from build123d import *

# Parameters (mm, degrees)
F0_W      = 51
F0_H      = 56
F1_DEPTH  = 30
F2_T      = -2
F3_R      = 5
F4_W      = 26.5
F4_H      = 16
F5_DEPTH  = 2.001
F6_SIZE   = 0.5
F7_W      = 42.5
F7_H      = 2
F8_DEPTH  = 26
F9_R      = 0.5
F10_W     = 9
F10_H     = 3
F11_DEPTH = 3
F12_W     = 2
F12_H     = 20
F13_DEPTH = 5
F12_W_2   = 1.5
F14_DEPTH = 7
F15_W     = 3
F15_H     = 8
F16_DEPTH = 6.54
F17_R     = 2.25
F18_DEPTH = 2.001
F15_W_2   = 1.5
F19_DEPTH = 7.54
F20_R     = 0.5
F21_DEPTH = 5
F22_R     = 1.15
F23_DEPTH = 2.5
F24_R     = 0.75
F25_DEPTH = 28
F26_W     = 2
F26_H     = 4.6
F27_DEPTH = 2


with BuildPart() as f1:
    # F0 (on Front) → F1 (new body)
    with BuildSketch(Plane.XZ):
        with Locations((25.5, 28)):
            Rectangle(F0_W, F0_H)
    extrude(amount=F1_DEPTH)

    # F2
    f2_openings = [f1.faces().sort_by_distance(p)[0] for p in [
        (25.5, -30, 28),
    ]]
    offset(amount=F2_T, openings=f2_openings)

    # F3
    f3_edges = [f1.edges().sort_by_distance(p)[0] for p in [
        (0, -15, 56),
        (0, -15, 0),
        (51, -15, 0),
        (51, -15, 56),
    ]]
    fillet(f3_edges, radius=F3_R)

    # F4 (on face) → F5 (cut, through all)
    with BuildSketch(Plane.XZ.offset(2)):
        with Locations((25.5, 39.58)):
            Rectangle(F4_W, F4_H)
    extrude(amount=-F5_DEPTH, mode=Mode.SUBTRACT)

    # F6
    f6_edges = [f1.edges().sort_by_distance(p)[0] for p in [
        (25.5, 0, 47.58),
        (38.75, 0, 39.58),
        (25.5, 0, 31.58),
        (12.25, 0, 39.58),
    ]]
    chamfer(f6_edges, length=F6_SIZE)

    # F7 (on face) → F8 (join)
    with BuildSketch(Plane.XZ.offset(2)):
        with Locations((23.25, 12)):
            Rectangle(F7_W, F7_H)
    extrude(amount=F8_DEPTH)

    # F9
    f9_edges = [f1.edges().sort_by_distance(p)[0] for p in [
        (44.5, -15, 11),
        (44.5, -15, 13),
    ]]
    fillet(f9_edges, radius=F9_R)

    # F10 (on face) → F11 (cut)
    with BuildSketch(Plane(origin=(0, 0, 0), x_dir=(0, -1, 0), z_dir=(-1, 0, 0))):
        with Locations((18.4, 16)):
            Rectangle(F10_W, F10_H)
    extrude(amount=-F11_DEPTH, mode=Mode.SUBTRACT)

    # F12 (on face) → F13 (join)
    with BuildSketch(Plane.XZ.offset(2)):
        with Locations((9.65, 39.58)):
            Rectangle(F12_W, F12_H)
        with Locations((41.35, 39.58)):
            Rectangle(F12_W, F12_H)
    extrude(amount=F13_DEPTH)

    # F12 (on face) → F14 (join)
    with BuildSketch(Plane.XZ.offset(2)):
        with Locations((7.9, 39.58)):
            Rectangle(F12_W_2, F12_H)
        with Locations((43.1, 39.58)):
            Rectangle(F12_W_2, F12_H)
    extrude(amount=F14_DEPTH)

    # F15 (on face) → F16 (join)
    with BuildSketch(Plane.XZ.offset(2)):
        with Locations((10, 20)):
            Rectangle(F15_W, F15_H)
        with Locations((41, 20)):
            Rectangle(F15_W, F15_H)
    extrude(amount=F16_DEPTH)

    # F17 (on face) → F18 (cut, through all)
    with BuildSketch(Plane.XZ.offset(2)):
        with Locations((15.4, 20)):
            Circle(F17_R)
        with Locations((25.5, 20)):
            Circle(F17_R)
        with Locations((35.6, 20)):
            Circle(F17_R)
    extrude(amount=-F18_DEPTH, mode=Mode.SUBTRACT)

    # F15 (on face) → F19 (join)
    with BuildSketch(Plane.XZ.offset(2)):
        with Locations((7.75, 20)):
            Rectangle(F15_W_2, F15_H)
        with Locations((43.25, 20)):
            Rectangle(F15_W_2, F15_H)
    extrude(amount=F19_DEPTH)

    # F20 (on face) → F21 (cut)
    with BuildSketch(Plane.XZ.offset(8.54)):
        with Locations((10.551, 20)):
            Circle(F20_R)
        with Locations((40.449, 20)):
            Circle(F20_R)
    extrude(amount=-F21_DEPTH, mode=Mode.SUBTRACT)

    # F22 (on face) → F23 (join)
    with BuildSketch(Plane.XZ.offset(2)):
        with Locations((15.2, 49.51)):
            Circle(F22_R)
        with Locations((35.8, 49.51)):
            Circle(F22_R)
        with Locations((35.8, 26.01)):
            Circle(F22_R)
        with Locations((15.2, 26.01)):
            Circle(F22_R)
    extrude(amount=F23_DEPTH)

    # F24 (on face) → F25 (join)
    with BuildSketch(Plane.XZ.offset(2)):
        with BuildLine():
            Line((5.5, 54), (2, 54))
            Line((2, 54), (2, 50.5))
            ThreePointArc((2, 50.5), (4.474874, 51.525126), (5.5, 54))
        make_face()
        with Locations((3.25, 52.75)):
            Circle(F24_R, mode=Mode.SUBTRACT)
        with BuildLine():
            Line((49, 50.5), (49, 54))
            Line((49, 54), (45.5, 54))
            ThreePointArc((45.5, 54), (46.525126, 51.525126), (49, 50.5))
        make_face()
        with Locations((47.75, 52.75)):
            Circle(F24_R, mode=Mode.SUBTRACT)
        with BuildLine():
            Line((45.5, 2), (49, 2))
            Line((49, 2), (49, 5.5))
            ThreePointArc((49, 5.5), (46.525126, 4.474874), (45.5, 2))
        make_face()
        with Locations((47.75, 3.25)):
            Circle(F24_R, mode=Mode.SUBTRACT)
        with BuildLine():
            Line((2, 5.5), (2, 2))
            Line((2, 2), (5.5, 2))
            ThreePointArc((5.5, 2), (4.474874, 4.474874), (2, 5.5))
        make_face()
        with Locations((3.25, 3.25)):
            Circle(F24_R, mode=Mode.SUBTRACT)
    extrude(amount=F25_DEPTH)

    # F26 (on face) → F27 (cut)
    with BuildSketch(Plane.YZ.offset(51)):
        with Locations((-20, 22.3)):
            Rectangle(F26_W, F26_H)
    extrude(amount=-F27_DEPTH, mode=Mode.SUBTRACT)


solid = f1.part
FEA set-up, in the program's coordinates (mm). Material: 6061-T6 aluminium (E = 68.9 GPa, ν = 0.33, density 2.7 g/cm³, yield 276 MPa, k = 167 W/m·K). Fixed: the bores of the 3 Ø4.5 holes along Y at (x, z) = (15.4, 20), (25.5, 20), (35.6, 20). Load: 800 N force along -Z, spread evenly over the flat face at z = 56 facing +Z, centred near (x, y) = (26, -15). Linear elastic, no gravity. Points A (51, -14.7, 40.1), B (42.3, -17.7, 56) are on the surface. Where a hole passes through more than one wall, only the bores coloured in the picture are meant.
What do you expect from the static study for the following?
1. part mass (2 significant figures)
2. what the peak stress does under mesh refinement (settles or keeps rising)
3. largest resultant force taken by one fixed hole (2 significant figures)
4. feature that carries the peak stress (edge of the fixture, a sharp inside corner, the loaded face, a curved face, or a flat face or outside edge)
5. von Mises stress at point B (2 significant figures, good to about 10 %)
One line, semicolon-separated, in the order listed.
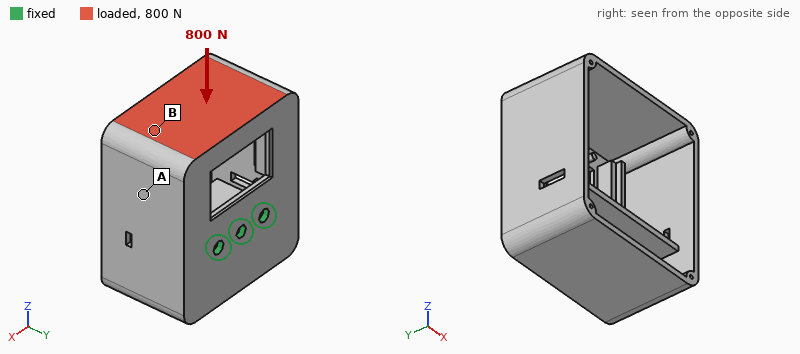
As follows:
54 g; keeps rising; 450 N; edge of the fixture; 38 MPa
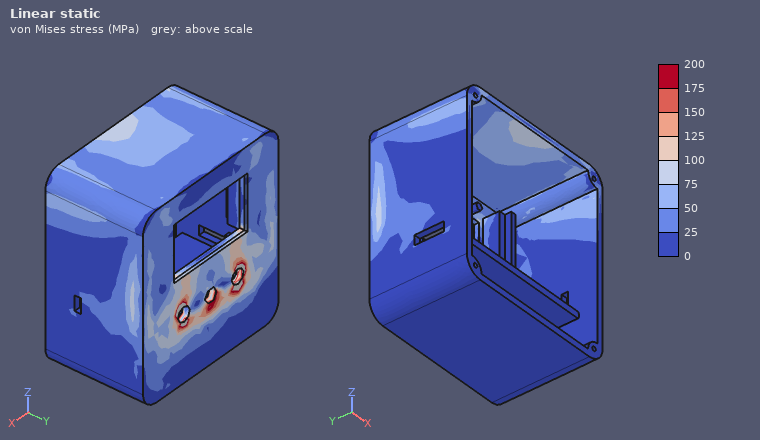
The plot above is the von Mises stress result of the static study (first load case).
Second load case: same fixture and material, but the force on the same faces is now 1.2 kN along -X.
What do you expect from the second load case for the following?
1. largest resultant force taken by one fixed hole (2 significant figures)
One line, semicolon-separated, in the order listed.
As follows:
1.8 kN
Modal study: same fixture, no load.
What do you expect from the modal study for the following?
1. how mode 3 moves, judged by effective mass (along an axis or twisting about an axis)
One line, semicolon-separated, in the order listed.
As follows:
along X
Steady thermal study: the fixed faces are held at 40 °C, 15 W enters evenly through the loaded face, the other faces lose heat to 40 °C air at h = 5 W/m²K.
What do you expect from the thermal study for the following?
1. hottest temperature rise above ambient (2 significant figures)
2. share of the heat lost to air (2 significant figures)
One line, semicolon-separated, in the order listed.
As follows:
30 K; 7.1 %
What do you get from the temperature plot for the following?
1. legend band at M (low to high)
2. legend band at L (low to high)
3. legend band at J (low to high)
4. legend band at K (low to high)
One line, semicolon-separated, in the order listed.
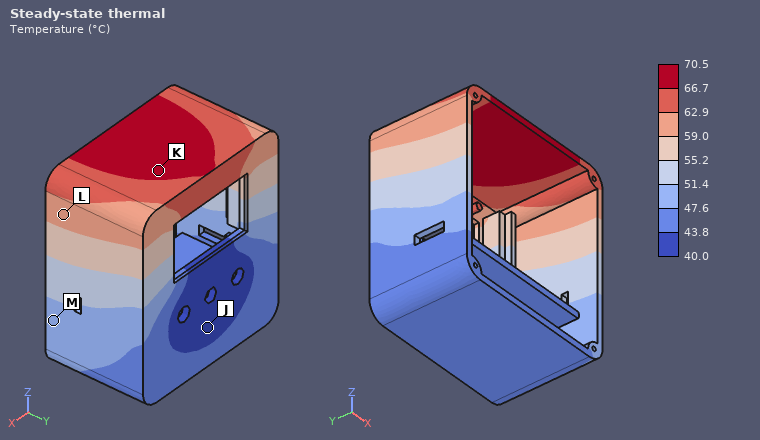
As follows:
47.6 to 51.4 °C; 59.0 to 62.9 °C; 40.0 to 43.8 °C; 66.7 to 70.5 °C
